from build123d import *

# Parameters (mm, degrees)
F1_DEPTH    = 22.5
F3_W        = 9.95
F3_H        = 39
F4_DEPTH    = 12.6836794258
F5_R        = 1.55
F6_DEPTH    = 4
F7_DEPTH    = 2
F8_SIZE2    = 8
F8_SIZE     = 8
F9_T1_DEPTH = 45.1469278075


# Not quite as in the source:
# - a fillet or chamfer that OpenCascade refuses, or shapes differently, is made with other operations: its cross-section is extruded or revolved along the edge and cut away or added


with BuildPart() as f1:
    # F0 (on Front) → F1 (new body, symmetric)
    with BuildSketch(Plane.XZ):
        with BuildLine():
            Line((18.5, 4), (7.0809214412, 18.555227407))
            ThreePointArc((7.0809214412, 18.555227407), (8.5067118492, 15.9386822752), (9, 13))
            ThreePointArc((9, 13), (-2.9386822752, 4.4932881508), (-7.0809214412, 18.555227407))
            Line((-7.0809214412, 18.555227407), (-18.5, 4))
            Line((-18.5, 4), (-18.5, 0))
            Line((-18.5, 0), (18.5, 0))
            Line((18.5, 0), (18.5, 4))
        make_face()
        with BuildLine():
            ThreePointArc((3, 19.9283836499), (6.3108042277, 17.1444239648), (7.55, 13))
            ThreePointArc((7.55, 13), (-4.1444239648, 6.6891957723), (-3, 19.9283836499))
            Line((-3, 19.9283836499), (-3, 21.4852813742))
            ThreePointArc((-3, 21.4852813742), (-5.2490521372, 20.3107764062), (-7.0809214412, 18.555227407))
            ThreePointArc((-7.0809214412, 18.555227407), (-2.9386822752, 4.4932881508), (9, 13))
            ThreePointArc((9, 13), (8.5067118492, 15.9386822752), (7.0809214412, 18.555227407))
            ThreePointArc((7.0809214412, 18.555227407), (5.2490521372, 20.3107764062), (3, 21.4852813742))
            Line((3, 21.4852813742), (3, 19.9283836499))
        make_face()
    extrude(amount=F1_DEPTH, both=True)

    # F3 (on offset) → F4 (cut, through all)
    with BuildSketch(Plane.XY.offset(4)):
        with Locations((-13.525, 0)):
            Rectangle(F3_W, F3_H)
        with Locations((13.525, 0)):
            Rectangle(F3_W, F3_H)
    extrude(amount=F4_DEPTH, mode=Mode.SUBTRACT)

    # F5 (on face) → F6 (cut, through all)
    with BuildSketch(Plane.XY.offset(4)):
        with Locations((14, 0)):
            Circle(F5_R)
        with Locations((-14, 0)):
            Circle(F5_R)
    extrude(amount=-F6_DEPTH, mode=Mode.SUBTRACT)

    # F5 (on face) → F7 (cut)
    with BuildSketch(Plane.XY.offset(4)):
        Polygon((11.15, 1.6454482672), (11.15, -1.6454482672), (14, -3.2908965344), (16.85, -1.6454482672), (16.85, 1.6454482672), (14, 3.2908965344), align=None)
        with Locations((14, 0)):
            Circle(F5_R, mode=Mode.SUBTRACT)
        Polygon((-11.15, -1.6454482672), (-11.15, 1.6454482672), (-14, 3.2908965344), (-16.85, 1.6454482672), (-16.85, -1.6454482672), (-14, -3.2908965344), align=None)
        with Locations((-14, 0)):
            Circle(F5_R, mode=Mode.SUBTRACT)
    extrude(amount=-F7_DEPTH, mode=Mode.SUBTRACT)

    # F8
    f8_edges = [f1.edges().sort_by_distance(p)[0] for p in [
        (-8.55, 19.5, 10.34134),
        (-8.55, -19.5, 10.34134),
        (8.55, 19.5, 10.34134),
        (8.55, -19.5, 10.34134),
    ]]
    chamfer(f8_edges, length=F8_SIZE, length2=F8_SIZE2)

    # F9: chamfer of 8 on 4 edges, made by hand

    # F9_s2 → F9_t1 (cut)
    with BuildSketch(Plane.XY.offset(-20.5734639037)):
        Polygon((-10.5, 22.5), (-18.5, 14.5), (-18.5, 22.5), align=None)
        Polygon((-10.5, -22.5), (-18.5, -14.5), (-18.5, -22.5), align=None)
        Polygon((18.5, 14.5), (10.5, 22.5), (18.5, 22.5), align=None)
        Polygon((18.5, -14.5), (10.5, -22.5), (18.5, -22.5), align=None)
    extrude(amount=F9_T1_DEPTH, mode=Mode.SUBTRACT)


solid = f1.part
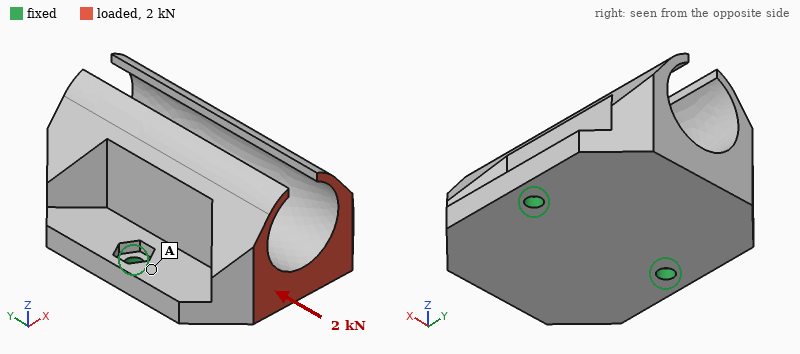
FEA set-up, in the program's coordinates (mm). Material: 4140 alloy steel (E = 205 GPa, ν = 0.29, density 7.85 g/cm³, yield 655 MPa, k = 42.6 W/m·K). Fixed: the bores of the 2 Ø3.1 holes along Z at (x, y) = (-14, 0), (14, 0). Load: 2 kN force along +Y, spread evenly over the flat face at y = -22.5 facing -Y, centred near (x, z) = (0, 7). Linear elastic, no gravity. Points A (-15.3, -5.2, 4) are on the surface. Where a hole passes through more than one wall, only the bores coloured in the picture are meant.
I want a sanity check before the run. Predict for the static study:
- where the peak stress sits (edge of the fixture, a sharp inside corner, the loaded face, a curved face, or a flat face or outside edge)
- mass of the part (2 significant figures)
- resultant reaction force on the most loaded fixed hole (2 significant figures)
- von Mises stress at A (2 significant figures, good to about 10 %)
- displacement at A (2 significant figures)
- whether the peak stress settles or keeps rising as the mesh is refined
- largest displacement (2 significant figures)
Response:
edge of the fixture
92 g
1.0 kN
59 MPa
16 µm
keeps rising
98 µm
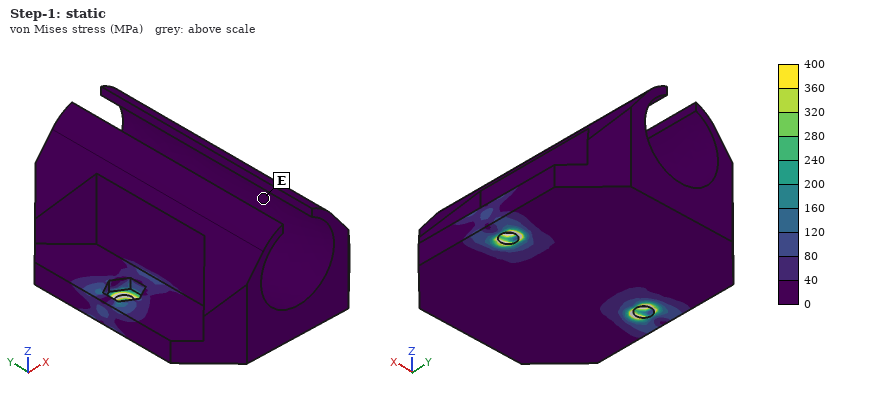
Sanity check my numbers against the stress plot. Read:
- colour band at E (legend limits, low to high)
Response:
0 to 40 MPa
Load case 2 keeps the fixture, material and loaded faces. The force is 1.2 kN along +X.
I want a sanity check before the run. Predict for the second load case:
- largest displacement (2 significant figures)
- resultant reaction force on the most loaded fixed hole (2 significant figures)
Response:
21 µm
1.1 kN
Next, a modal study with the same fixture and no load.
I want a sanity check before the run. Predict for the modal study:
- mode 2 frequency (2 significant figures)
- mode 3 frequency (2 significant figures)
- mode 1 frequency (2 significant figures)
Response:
8700 Hz
9000 Hz
2100 Hz
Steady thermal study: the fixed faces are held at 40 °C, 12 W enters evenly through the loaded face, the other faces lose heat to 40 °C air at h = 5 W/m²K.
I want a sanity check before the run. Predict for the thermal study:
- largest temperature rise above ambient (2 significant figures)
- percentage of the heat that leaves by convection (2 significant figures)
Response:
43 K
5.9 %
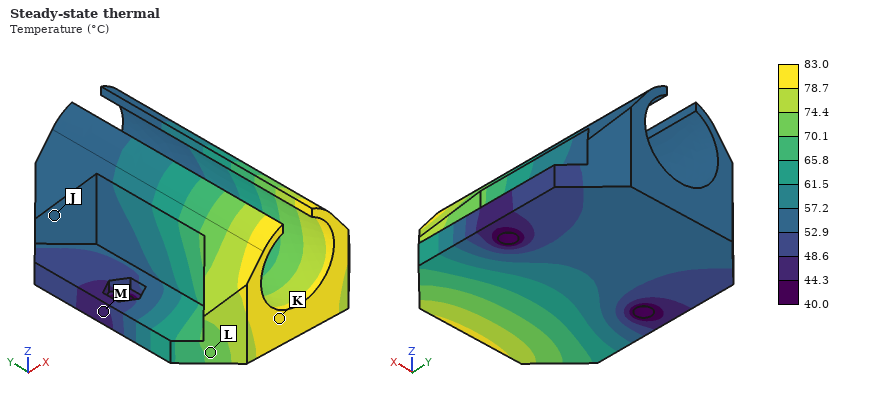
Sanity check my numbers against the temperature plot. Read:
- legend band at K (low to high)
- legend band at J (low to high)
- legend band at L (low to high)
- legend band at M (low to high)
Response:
78.7 to 83.0 °C
52.9 to 57.2 °C
70.1 to 74.4 °C
44.3 to 48.6 °C
